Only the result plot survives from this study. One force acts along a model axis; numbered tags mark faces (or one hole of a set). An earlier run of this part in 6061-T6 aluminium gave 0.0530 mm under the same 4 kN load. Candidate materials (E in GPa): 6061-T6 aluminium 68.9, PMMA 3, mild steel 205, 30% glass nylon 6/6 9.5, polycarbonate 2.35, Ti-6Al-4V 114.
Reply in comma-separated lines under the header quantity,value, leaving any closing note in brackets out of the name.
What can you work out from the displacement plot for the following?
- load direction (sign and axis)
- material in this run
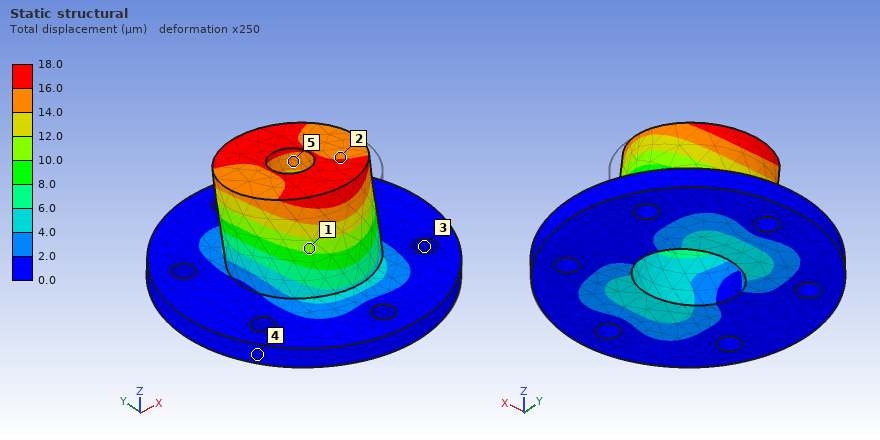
quantity,value
load direction,+Y
material in this run,mild steel
